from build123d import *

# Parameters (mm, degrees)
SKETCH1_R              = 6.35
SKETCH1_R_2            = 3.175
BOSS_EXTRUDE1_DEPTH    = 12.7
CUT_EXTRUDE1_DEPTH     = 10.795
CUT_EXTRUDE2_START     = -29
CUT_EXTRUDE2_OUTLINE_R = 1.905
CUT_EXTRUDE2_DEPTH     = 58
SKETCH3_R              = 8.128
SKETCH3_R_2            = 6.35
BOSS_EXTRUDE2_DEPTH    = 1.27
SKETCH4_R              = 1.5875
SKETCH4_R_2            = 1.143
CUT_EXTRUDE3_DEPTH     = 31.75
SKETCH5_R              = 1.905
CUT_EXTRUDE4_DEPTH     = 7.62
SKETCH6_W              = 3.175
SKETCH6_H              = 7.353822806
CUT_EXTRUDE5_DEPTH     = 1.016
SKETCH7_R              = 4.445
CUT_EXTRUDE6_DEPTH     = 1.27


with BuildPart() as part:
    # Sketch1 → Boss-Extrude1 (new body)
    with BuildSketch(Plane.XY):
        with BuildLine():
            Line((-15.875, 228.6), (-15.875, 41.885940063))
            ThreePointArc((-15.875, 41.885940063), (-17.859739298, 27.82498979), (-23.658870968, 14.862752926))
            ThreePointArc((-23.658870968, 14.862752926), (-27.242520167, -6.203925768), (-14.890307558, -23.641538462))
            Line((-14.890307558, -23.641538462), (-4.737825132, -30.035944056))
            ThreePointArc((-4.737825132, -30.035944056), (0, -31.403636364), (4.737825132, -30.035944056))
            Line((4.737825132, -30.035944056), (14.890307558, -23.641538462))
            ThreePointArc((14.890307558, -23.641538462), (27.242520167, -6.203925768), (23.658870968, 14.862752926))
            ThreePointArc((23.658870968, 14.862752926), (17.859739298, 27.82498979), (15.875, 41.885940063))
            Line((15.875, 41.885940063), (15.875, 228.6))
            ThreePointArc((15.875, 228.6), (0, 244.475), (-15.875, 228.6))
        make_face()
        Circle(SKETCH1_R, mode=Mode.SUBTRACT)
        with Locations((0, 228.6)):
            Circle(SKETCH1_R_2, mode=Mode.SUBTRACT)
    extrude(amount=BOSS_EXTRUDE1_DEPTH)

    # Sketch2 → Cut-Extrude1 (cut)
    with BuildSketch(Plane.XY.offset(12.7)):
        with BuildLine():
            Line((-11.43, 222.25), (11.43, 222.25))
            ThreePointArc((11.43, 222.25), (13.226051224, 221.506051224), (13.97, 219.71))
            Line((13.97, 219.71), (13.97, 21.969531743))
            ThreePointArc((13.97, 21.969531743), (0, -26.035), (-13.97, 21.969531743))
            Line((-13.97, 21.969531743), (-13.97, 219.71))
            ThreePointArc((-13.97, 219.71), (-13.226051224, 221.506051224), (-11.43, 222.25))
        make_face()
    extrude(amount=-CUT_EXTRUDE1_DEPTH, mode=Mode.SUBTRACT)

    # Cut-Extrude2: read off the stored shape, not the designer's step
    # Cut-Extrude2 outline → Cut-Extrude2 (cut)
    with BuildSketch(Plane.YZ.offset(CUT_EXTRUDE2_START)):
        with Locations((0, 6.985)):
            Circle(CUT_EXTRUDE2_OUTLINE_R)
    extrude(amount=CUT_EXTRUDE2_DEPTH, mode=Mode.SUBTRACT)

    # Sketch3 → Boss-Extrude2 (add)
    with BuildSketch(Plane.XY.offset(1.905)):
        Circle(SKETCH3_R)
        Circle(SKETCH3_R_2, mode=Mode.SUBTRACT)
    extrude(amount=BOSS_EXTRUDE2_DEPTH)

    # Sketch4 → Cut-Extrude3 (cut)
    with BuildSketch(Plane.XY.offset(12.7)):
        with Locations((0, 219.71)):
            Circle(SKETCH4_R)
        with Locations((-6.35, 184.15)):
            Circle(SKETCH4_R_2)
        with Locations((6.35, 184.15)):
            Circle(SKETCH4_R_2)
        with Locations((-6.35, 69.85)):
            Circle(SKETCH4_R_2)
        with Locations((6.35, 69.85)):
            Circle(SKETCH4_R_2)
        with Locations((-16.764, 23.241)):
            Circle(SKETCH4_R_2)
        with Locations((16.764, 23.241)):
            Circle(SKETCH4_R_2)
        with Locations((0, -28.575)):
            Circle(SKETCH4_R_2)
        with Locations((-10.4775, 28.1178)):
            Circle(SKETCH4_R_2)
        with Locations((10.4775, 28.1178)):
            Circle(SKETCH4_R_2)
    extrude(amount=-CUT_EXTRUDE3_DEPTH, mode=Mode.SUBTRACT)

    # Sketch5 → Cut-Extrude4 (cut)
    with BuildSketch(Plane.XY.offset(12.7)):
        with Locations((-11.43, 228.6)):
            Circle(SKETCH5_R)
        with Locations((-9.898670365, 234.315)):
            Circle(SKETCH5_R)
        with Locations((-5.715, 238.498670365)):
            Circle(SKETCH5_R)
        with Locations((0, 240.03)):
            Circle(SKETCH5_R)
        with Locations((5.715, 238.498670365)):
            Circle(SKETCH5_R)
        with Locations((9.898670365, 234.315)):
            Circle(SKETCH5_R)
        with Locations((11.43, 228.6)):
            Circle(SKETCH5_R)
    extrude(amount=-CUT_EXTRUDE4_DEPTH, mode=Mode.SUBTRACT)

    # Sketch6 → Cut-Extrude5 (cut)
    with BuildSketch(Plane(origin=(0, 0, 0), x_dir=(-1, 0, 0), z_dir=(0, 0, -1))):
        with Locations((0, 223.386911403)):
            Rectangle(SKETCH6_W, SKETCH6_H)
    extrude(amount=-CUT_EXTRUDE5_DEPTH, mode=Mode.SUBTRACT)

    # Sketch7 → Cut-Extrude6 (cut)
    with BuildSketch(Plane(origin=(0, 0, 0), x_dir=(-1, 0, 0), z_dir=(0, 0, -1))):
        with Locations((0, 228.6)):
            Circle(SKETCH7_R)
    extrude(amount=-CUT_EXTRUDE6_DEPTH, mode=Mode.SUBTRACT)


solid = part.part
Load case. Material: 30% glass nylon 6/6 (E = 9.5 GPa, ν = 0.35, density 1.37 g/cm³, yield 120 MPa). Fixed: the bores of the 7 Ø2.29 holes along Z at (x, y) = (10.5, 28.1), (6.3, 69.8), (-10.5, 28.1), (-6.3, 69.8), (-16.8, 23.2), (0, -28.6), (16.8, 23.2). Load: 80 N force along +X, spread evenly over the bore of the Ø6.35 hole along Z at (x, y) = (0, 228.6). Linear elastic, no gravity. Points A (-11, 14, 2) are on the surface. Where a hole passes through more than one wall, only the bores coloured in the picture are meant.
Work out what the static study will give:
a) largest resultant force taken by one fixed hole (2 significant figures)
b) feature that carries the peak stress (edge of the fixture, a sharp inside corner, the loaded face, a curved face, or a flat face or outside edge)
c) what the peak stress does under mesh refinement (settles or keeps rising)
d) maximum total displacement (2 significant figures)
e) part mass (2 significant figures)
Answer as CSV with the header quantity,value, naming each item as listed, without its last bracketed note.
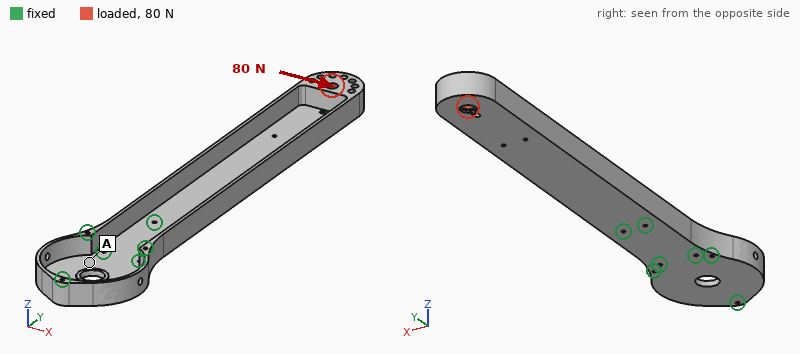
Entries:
quantity,value
largest resultant force taken by one fixed hole,430 N
feature that carries the peak stress,edge of the fixture
what the peak stress does under mesh refinement,keeps rising
maximum total displacement,3.0 mm
part mass,48 g
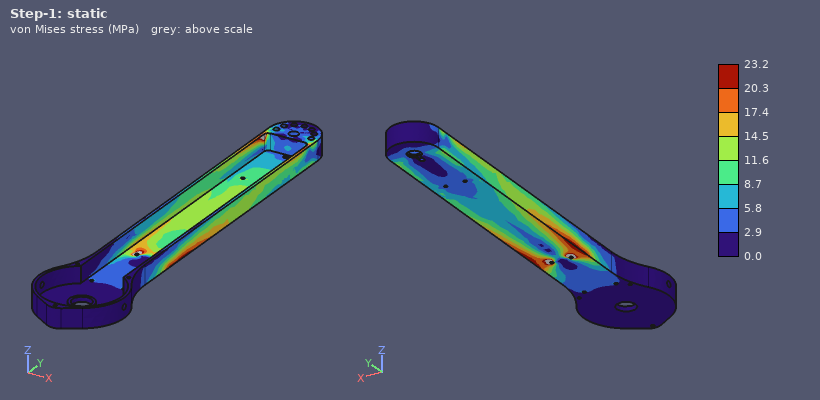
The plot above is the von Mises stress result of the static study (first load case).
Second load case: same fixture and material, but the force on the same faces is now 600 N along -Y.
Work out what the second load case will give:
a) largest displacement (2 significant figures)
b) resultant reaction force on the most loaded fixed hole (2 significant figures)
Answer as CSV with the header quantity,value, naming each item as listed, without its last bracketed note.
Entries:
quantity,value
largest displacement,3.1 mm
resultant reaction force on the most loaded fixed hole,140 N
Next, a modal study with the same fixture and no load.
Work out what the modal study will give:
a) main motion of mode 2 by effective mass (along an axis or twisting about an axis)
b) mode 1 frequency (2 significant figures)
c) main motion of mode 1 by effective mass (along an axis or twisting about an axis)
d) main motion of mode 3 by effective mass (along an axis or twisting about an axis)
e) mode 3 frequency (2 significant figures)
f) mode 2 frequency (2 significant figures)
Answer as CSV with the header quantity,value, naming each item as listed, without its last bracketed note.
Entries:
quantity,value
main motion of mode 2 by effective mass,along X
mode 1 frequency,110 Hz
main motion of mode 1 by effective mass,along Z
main motion of mode 3 by effective mass,along X
mode 3 frequency,430 Hz
mode 2 frequency,230 Hz
